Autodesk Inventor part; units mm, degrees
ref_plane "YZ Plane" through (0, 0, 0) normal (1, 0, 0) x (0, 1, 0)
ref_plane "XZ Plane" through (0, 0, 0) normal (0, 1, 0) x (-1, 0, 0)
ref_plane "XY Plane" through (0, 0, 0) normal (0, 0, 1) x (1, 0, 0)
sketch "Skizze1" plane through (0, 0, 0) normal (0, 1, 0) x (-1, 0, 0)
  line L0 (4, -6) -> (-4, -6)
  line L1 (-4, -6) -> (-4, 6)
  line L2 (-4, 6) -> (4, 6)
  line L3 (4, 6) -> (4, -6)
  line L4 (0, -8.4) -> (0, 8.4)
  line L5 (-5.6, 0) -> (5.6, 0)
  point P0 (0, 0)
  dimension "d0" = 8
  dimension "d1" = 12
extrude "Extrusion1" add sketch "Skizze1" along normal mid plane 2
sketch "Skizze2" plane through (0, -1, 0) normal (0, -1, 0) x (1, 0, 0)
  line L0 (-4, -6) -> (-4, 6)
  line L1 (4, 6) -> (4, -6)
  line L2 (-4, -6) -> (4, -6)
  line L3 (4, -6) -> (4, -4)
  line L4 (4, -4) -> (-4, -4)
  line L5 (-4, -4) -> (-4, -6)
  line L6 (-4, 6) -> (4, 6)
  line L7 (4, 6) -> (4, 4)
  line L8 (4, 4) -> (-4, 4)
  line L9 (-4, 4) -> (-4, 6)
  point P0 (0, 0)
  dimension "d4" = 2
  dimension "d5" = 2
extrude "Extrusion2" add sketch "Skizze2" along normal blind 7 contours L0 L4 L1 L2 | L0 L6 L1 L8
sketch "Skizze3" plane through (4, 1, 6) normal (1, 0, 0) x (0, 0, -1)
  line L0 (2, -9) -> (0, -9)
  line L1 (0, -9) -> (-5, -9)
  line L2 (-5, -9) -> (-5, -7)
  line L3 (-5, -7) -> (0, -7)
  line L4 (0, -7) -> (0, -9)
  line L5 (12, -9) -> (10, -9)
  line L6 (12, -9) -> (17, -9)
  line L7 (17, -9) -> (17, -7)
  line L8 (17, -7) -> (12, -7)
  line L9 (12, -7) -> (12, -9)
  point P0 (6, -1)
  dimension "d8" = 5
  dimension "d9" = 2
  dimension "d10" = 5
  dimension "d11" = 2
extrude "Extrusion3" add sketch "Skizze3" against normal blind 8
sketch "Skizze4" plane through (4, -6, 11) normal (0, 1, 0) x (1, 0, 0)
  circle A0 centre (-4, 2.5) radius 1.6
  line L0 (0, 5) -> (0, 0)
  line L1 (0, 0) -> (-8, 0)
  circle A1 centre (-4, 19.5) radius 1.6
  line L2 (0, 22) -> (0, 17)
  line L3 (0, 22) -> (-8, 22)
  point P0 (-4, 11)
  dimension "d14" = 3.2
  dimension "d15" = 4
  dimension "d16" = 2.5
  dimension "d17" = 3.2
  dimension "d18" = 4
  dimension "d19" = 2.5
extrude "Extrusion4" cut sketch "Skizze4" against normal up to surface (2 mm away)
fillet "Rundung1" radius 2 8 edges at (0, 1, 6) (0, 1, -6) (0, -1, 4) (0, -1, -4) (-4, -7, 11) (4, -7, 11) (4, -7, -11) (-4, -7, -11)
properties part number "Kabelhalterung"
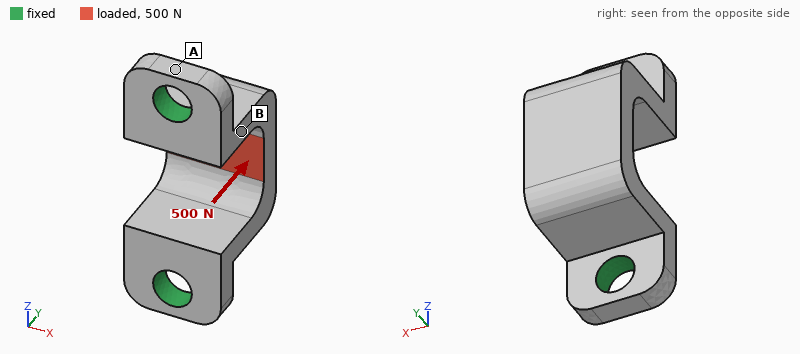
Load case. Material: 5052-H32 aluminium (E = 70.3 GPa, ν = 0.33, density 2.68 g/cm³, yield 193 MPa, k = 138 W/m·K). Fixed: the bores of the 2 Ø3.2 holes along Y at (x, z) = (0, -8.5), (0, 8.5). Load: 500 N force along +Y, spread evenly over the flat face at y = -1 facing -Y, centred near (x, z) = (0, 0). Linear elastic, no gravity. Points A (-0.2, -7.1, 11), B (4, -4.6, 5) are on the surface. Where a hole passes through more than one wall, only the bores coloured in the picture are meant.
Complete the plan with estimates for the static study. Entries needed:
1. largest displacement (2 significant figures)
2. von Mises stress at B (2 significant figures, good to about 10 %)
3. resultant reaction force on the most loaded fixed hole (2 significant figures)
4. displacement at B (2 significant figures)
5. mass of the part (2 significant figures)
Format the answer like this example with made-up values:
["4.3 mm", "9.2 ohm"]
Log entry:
["11 µm", "29 MPa", "290 N", "2.9 µm", "1.4 g"]
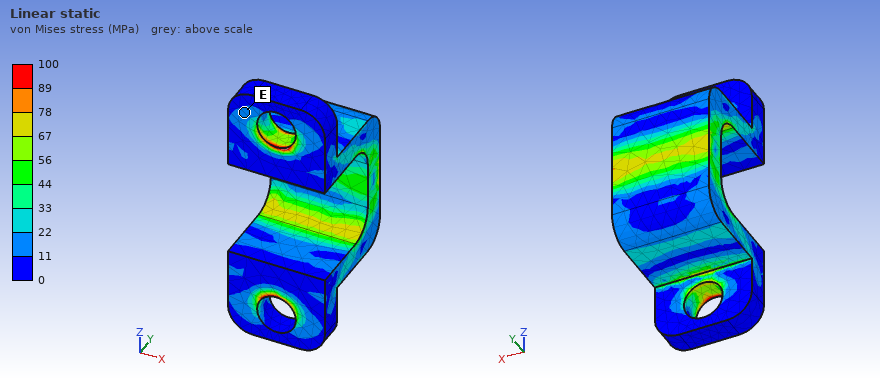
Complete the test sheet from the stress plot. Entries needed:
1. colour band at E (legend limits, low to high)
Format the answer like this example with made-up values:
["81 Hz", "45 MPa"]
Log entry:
["11 to 22 MPa"]
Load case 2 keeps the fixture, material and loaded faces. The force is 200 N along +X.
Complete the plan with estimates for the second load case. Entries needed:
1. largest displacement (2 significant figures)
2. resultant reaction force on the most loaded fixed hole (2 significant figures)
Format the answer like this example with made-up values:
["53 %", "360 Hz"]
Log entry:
["19 µm", "100 N"]
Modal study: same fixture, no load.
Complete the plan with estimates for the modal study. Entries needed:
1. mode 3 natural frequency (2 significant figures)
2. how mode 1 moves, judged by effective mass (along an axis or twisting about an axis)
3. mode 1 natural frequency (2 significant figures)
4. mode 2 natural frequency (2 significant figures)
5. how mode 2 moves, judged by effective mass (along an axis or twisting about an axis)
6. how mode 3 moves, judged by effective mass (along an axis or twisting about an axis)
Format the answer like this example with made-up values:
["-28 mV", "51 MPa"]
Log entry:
["34 kHz", "along X", "20 kHz", "28 kHz", "along Z", "twisting about Y"]
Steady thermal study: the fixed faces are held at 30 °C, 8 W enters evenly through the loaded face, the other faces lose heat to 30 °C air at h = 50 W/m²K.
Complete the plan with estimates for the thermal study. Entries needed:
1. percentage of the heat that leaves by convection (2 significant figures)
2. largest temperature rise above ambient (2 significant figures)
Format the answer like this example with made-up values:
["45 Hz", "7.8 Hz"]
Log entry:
["3.3 %", "21 K"]
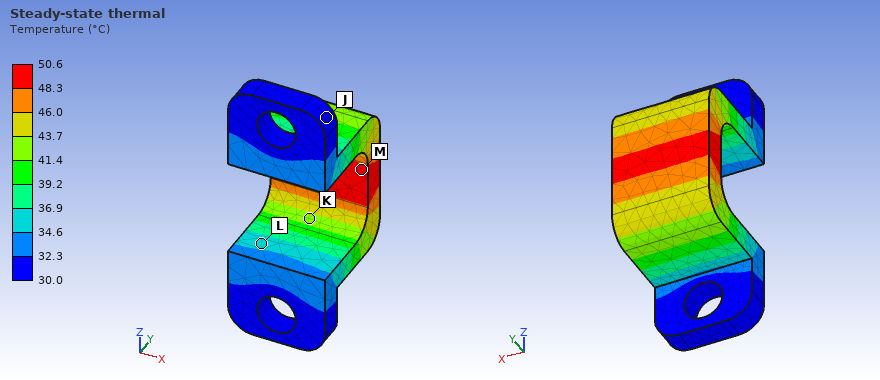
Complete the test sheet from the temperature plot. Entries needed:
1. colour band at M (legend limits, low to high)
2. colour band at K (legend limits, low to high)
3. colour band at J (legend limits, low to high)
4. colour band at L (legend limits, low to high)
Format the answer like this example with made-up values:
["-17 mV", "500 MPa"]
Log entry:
["48.3 to 50.6 °C", "41.4 to 43.7 °C", "30.0 to 32.3 °C", "34.6 to 36.9 °C"]
